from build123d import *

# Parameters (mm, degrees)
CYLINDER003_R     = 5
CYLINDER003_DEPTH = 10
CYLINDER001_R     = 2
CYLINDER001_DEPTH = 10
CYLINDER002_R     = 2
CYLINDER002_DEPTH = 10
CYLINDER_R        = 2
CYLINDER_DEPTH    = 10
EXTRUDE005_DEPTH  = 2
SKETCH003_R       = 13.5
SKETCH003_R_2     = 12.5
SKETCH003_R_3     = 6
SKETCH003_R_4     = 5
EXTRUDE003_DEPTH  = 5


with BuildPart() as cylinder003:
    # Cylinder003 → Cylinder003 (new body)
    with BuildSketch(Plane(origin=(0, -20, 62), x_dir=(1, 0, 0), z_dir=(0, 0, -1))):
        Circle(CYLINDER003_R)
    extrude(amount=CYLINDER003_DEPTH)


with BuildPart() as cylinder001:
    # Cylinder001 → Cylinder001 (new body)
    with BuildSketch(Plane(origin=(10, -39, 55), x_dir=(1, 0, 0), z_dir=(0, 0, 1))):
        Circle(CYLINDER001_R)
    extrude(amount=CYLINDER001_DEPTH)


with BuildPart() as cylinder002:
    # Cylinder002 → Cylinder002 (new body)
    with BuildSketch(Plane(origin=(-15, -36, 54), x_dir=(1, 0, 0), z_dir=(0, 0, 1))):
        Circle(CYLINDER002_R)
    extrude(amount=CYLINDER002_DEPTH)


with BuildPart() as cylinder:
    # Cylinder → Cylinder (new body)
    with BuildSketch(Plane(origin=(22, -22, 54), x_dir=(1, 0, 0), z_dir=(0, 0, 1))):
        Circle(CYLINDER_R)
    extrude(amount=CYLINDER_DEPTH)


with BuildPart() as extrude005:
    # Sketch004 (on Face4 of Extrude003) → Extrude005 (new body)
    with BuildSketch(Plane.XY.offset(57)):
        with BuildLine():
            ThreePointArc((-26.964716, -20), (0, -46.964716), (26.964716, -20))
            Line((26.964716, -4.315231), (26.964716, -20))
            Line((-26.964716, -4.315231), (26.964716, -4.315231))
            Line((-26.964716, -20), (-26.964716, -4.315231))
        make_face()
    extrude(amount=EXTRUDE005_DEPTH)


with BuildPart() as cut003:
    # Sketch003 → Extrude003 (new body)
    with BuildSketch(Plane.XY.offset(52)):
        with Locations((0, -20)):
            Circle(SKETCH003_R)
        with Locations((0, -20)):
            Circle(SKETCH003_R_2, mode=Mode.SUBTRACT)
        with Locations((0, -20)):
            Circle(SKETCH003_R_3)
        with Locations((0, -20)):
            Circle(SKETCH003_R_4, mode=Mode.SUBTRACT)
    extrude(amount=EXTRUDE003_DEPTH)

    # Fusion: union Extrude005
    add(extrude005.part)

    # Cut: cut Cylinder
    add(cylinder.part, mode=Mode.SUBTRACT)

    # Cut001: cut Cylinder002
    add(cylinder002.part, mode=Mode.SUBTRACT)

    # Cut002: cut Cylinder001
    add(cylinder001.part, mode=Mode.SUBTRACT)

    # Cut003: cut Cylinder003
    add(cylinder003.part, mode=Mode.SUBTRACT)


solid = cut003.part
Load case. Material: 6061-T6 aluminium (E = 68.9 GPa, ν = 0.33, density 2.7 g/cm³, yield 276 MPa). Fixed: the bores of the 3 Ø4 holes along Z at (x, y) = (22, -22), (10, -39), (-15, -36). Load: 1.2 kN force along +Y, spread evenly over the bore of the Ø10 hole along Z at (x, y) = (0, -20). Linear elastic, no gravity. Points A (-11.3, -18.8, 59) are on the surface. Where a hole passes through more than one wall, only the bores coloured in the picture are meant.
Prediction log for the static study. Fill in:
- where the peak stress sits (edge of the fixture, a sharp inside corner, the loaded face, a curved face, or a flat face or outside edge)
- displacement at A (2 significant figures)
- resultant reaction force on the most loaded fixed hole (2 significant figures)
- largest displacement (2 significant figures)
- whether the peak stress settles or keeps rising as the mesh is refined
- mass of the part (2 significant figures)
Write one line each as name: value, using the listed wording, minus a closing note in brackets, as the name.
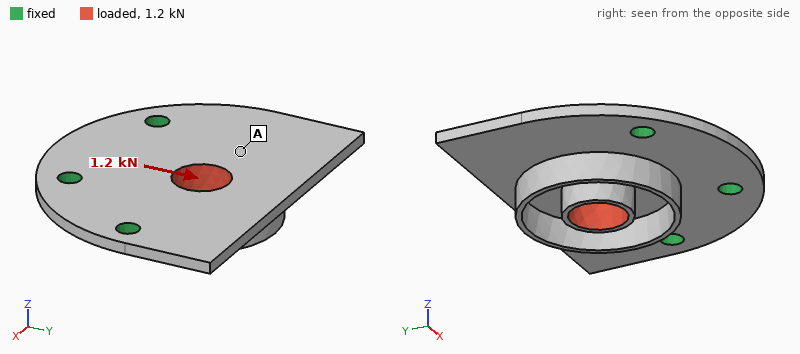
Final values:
where the peak stress sits: edge of the fixture
displacement at A: 0.096 mm
resultant reaction force on the most loaded fixed hole: 560 N
largest displacement: 0.23 mm
whether the peak stress settles or keeps rising as the mesh is refined: keeps rising
mass of the part: 12 g
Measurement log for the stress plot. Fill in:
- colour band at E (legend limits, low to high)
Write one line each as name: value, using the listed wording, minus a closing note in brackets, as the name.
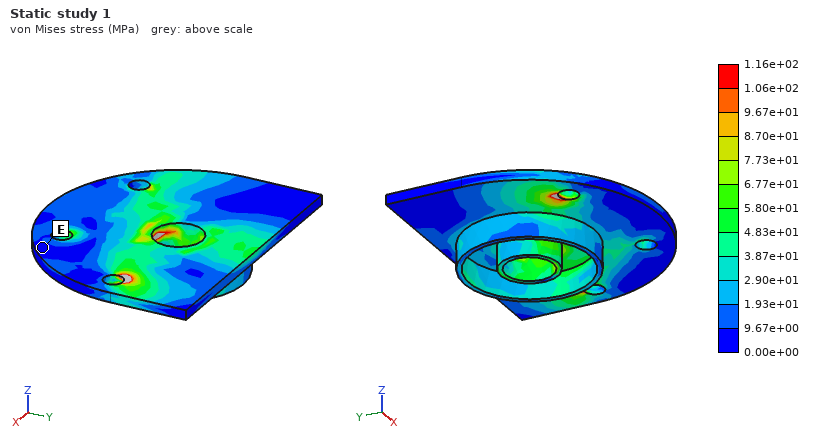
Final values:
colour band at E: 0.00e+00 to 9.67e+00 MPa
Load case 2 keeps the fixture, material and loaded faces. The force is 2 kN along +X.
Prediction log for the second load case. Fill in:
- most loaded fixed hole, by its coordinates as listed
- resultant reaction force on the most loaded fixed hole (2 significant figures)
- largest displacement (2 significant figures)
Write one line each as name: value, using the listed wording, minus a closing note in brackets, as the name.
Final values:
most loaded fixed hole, by its coordinates as listed: (22, -22)
resultant reaction force on the most loaded fixed hole: 1.1 kN
largest displacement: 0.22 mm
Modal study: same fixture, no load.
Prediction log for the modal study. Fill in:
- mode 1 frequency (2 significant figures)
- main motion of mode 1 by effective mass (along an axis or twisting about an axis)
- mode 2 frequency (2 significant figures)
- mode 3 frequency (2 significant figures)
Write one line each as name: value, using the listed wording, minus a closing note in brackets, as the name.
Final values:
mode 1 frequency: 2200 Hz
main motion of mode 1 by effective mass: along Z
mode 2 frequency: 4900 Hz
mode 3 frequency: 8500 Hz
